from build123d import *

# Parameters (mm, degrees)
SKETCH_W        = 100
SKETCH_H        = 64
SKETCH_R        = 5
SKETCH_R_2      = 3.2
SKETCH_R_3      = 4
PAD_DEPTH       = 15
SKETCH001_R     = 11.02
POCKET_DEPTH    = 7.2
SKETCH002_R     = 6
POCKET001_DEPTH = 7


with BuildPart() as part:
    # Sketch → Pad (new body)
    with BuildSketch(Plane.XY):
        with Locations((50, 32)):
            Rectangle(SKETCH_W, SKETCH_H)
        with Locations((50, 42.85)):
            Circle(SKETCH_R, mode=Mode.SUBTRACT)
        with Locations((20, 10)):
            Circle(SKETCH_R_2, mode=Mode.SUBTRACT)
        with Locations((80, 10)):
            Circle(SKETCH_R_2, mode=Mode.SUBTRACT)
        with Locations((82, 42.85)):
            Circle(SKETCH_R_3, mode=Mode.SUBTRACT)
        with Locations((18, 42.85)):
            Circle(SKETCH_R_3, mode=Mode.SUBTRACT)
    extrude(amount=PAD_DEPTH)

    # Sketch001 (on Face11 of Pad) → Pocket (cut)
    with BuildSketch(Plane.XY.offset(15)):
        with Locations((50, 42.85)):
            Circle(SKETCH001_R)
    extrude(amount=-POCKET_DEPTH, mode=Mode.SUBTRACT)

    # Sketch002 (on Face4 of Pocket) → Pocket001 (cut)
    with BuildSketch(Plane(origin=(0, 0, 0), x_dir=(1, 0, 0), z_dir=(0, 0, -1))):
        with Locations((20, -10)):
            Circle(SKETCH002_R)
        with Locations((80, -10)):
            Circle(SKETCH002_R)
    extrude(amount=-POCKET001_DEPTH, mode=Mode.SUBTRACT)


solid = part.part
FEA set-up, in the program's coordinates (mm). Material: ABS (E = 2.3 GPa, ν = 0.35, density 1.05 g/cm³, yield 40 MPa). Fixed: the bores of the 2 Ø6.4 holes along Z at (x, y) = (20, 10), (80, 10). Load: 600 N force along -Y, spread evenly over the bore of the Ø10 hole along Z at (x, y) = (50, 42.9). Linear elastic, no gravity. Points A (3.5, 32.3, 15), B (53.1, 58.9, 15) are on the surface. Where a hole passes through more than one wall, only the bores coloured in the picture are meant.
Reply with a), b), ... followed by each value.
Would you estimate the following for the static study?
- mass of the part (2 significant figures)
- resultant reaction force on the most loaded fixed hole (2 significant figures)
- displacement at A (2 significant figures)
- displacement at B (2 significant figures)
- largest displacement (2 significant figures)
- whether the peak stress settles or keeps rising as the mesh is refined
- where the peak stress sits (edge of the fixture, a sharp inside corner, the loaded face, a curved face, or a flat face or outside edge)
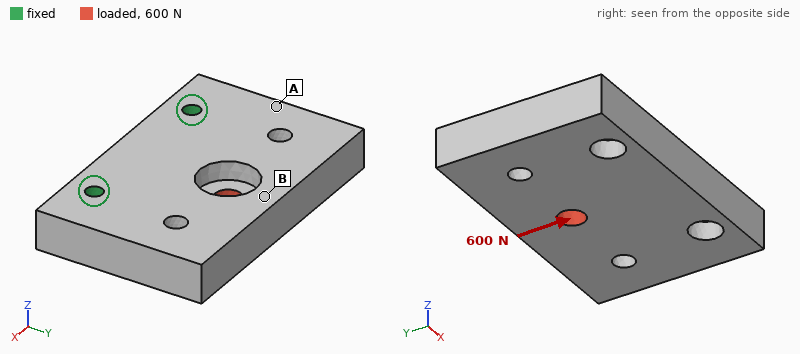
a) 93 g
b) 310 N
c) 0.061 mm
d) 0.18 mm
e) 0.21 mm
f) keeps rising
g) edge of the fixture
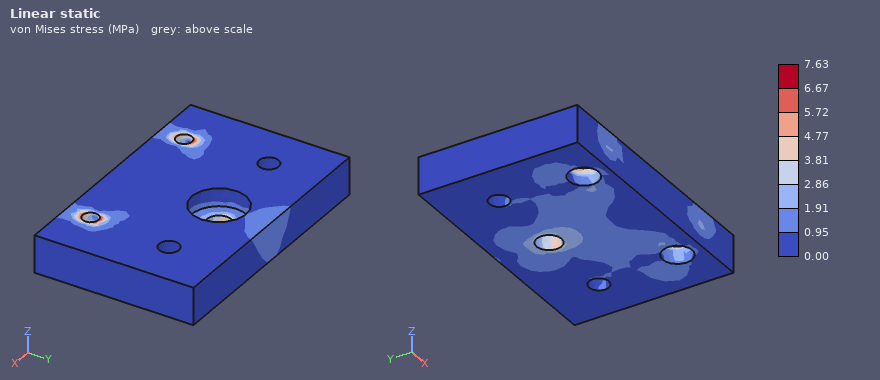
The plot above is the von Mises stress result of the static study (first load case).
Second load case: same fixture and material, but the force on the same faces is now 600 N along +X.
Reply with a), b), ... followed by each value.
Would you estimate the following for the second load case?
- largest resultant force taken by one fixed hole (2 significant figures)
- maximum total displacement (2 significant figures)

a) 440 N
b) 58 µm
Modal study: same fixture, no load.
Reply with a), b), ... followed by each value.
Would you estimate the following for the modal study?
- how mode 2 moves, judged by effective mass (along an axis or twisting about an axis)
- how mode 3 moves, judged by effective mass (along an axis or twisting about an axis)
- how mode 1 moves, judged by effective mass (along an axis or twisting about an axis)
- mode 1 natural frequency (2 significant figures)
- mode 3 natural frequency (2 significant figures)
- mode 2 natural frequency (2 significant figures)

a) twisting about Y
b) along X
c) along Z
d) 620 Hz
e) 2300 Hz
f) 1300 Hz
